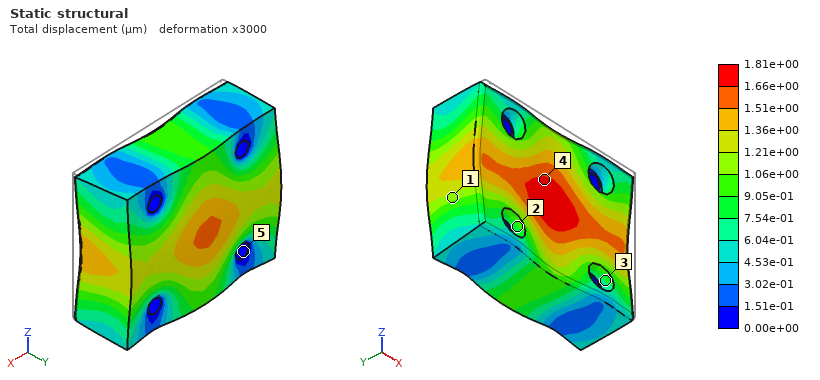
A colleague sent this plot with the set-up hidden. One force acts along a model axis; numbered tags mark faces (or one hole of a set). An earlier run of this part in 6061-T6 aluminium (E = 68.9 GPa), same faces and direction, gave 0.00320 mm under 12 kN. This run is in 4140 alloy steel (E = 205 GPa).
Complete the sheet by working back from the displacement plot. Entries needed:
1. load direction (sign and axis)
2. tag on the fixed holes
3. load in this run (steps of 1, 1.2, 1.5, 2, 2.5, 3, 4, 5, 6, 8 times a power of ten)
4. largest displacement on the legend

+Y
5
20 kN
1.81e+00 µm
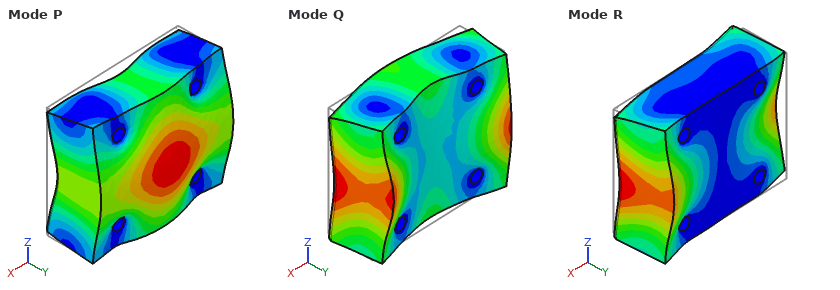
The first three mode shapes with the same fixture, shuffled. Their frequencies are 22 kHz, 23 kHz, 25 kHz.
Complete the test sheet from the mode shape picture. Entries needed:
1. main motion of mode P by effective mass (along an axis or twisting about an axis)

along Y
